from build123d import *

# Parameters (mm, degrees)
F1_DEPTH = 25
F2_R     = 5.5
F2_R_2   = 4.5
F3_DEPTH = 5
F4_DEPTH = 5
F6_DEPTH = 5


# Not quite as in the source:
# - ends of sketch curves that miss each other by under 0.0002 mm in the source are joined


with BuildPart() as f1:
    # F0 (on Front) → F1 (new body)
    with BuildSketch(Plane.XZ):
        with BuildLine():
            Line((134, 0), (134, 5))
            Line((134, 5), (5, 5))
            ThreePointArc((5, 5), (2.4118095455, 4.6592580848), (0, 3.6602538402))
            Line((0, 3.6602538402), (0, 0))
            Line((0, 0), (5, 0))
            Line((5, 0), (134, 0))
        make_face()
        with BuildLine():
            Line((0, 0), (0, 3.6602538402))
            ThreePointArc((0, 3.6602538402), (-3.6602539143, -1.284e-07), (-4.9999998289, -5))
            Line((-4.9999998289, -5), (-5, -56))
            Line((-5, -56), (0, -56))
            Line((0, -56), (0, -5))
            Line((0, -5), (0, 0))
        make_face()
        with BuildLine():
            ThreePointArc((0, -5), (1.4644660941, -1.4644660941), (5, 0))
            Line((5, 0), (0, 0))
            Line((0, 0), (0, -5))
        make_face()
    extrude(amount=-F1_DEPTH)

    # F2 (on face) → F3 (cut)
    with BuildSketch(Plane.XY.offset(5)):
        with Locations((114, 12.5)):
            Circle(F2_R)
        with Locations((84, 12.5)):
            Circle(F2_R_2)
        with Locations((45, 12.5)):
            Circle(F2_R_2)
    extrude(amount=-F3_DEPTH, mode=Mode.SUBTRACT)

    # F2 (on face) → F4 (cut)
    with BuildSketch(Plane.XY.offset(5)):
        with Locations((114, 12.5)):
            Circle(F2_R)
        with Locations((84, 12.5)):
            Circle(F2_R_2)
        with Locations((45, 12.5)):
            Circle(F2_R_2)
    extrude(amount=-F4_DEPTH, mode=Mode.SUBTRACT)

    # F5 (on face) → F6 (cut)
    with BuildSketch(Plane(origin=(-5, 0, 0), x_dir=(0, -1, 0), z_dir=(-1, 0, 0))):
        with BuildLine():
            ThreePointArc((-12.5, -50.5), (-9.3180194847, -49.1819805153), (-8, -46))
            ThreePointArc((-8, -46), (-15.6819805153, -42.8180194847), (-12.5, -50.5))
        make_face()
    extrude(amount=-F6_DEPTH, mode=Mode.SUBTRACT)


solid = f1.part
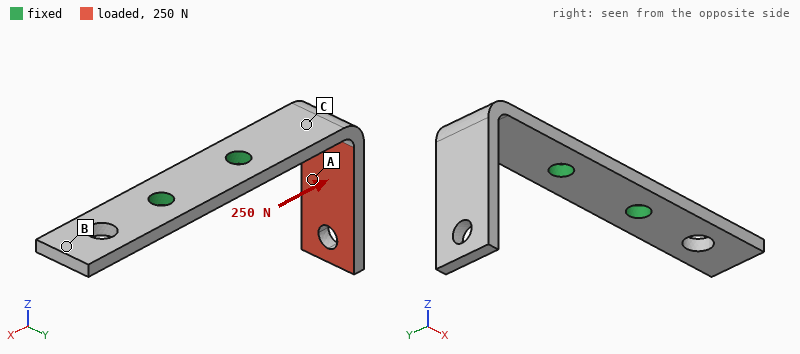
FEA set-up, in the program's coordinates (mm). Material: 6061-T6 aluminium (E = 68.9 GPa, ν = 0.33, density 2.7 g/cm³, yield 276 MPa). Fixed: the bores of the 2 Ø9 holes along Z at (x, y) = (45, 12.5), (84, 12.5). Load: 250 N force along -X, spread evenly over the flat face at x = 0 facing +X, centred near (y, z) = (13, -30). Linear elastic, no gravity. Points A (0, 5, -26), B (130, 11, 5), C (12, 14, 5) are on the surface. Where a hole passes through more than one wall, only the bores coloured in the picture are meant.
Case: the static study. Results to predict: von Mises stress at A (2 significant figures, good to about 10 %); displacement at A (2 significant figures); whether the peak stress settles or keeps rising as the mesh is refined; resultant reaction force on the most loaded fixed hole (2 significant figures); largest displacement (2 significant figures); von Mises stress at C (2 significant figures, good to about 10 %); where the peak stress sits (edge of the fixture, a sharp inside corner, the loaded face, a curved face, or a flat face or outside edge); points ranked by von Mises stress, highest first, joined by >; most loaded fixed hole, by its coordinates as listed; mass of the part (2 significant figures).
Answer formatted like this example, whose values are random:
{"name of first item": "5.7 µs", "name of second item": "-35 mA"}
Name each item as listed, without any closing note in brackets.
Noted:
{"von Mises stress at A": "21 MPa", "displacement at A": "0.74 mm", "whether the peak stress settles or keeps rising as the mesh is refined": "keeps rising", "resultant reaction force on the most loaded fixed hole": "230 N", "largest displacement": "1.5 mm", "von Mises stress at C": "69 MPa", "where the peak stress sits": "edge of the fixture", "points ranked by von Mises stress, highest first, joined by >": "C > A > B", "most loaded fixed hole, by its coordinates as listed": "(45, 12.5)", "mass of the part": "61 g"}
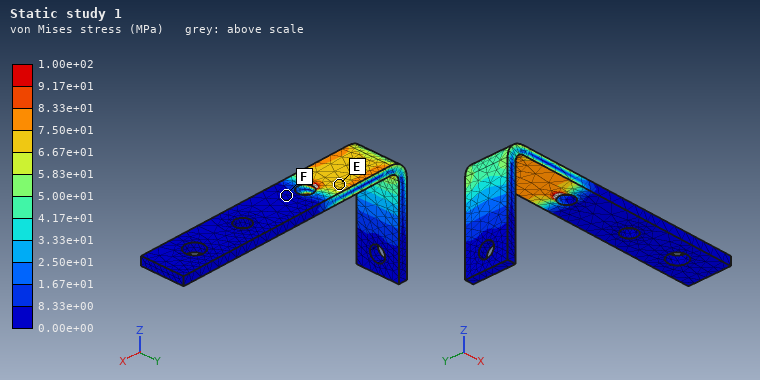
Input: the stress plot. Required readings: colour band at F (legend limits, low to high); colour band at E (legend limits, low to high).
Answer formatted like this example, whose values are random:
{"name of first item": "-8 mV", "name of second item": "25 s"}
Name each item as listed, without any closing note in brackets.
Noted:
{"colour band at F": "0.00e+00 to 8.33e+00 MPa", "colour band at E": "6.67e+01 to 7.50e+01 MPa"}
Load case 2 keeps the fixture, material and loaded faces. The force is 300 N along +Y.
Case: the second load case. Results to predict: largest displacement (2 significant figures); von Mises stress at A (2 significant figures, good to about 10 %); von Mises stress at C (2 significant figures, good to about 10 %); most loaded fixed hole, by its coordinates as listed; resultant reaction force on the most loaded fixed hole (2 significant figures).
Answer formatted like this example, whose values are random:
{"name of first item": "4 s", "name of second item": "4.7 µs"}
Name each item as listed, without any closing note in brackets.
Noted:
{"largest displacement": "1.0 mm", "von Mises stress at A": "8.5 MPa", "von Mises stress at C": "80 MPa", "most loaded fixed hole, by its coordinates as listed": "(45, 12.5)", "resultant reaction force on the most loaded fixed hole": "440 N"}
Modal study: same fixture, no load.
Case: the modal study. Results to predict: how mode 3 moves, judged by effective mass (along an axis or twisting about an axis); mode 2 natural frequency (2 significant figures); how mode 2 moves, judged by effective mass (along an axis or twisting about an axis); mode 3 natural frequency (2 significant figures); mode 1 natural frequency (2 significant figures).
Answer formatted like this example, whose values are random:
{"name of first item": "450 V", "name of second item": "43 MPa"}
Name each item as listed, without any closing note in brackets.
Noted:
{"how mode 3 moves, judged by effective mass": "along Z", "mode 2 natural frequency": "820 Hz", "how mode 2 moves, judged by effective mass": "along Y", "mode 3 natural frequency": "1600 Hz", "mode 1 natural frequency": "540 Hz"}
